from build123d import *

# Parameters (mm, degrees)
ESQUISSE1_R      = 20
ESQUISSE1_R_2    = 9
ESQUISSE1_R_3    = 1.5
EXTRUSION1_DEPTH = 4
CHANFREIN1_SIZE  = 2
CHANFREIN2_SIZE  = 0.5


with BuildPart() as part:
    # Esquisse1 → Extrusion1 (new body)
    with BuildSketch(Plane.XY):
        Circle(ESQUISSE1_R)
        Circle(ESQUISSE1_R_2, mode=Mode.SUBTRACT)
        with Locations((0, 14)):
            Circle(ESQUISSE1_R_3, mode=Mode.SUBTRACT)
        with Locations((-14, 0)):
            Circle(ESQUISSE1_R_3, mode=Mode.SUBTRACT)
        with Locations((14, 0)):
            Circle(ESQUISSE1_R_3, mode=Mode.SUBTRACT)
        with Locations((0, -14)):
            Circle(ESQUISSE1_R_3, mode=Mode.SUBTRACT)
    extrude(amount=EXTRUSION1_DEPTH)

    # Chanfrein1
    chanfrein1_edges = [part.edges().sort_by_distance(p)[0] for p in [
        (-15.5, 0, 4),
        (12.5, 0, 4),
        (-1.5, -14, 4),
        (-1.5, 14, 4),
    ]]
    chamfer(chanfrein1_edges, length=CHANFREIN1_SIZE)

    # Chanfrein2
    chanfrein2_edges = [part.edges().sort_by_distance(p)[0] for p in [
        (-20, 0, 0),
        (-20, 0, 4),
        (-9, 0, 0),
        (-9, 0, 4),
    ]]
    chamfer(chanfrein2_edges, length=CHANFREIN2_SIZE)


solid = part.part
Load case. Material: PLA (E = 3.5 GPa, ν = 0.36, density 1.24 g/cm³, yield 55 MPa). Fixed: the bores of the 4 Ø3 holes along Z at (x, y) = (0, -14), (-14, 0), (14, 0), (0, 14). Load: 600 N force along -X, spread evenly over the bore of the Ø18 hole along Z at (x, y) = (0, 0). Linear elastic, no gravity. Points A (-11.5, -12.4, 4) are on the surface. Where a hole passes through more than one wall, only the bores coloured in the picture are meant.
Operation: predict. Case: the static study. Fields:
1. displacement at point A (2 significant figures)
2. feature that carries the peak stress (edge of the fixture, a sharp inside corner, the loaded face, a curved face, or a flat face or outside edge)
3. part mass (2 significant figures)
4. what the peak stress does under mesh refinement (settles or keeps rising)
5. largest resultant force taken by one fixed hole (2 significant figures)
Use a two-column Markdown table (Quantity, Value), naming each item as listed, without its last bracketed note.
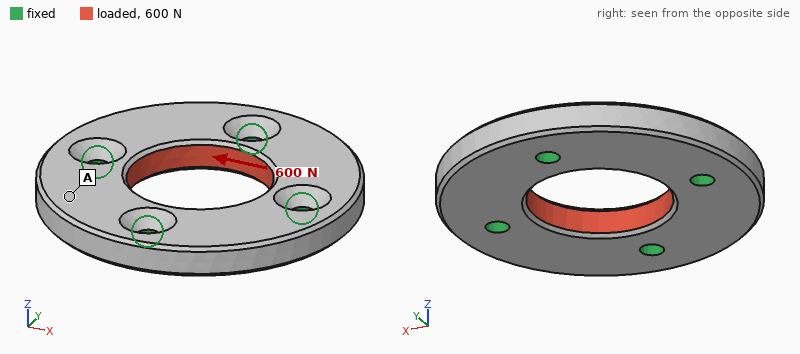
| Quantity | Value |
|---|---|
| displacement at point A | 16 µm |
| feature that carries the peak stress | edge of the fixture |
| part mass | 4.6 g |
| what the peak stress does under mesh refinement | keeps rising |
| largest resultant force taken by one fixed hole | 150 N |
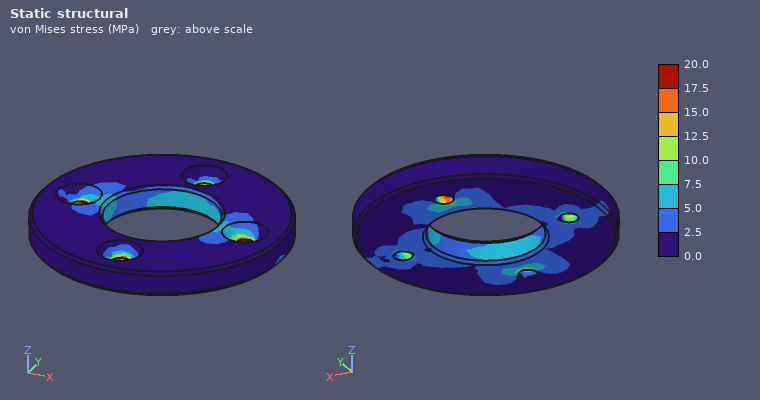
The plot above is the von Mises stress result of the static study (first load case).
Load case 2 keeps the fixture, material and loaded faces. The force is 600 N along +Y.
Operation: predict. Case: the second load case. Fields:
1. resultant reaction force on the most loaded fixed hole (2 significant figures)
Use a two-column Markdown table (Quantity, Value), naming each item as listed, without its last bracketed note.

| Quantity | Value |
|---|---|
| resultant reaction force on the most loaded fixed hole | 150 N |
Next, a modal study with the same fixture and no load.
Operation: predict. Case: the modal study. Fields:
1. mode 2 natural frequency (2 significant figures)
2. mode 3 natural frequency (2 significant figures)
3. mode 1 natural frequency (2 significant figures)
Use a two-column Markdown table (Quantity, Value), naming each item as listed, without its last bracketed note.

| Quantity | Value |
|---|---|
| mode 2 natural frequency | 6900 Hz |
| mode 3 natural frequency | 6900 Hz |
| mode 1 natural frequency | 6000 Hz |
